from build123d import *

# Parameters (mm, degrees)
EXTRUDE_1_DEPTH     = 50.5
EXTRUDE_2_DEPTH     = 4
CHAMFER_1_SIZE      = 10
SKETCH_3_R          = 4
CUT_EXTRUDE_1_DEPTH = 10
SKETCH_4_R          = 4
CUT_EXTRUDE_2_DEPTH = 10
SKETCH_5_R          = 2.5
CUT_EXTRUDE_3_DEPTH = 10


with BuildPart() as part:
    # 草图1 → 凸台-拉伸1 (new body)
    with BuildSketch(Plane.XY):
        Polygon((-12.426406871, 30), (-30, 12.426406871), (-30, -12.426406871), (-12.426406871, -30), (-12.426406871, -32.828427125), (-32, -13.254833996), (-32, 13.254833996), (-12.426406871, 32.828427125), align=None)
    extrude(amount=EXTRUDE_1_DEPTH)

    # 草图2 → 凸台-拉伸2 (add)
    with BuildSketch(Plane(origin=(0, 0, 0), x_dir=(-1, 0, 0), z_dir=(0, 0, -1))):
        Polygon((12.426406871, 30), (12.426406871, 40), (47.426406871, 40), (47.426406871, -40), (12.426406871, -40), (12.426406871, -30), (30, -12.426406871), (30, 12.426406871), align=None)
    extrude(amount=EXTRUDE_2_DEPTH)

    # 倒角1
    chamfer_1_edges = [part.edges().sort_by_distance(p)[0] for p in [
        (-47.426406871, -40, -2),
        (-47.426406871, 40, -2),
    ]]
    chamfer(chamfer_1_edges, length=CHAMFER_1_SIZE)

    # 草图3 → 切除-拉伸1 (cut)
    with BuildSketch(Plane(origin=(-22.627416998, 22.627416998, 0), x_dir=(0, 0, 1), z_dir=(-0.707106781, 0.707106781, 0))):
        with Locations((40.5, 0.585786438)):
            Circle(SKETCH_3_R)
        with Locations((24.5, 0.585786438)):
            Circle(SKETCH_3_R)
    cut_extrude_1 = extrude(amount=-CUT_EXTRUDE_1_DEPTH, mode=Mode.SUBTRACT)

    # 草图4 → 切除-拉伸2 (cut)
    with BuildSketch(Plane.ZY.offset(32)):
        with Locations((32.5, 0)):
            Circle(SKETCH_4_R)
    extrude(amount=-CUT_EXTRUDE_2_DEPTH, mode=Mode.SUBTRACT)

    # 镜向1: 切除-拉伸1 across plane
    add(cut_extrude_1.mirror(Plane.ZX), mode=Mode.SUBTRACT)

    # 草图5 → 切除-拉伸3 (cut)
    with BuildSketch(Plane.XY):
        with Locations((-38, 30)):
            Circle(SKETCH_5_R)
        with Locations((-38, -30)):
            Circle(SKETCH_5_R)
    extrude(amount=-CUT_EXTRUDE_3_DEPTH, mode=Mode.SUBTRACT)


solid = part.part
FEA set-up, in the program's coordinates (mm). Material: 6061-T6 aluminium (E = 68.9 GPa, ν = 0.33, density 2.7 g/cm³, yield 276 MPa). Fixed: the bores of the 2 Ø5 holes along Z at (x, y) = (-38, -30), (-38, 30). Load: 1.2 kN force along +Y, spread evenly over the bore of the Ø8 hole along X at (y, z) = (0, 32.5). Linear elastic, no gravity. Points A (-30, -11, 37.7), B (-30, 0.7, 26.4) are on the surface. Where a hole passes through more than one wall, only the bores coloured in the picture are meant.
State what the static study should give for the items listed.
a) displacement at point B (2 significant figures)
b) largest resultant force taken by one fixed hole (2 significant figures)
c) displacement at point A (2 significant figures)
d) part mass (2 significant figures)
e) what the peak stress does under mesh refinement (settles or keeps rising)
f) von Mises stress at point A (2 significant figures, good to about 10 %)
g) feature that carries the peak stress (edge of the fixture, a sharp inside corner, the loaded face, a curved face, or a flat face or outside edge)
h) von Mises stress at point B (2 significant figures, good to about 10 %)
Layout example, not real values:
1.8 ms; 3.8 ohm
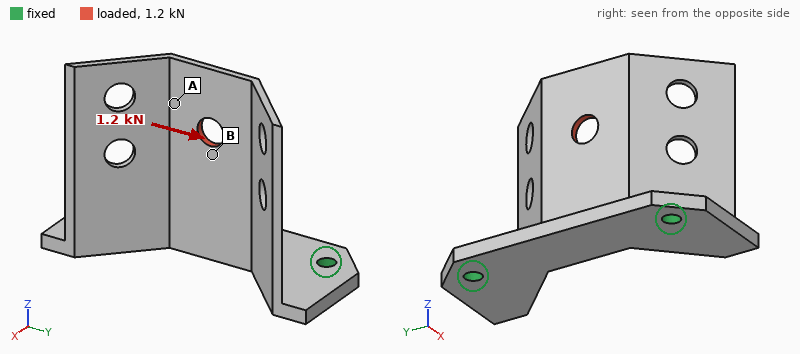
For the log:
0.15 mm; 1.1 kN; 0.23 mm; 41 g; keeps rising; 33 MPa; edge of the fixture; 80 MPa
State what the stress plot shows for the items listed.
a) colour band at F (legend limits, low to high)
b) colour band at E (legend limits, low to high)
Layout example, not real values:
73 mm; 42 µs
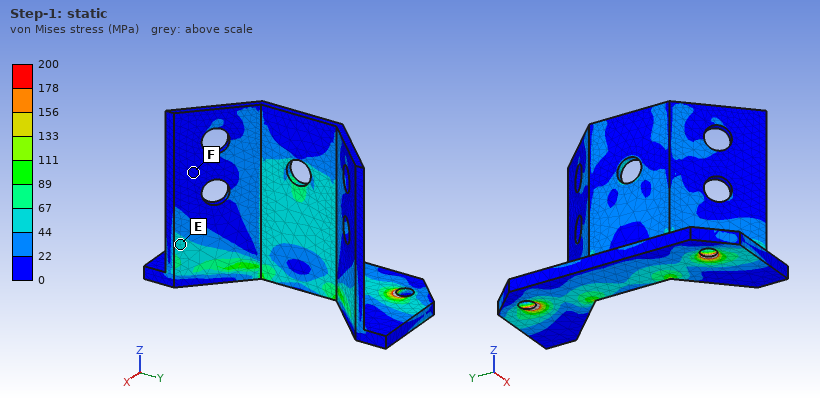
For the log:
0 to 22 MPa; 44 to 67 MPa
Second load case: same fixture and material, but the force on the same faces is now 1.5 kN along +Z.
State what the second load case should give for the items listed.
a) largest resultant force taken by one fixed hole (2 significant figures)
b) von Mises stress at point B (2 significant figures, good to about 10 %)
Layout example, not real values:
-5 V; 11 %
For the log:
830 N; 30 MPa
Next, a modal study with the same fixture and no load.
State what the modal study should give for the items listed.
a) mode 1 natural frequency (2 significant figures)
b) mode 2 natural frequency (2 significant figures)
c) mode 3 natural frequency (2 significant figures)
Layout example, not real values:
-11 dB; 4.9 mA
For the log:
1300 Hz; 1300 Hz; 2300 Hz
